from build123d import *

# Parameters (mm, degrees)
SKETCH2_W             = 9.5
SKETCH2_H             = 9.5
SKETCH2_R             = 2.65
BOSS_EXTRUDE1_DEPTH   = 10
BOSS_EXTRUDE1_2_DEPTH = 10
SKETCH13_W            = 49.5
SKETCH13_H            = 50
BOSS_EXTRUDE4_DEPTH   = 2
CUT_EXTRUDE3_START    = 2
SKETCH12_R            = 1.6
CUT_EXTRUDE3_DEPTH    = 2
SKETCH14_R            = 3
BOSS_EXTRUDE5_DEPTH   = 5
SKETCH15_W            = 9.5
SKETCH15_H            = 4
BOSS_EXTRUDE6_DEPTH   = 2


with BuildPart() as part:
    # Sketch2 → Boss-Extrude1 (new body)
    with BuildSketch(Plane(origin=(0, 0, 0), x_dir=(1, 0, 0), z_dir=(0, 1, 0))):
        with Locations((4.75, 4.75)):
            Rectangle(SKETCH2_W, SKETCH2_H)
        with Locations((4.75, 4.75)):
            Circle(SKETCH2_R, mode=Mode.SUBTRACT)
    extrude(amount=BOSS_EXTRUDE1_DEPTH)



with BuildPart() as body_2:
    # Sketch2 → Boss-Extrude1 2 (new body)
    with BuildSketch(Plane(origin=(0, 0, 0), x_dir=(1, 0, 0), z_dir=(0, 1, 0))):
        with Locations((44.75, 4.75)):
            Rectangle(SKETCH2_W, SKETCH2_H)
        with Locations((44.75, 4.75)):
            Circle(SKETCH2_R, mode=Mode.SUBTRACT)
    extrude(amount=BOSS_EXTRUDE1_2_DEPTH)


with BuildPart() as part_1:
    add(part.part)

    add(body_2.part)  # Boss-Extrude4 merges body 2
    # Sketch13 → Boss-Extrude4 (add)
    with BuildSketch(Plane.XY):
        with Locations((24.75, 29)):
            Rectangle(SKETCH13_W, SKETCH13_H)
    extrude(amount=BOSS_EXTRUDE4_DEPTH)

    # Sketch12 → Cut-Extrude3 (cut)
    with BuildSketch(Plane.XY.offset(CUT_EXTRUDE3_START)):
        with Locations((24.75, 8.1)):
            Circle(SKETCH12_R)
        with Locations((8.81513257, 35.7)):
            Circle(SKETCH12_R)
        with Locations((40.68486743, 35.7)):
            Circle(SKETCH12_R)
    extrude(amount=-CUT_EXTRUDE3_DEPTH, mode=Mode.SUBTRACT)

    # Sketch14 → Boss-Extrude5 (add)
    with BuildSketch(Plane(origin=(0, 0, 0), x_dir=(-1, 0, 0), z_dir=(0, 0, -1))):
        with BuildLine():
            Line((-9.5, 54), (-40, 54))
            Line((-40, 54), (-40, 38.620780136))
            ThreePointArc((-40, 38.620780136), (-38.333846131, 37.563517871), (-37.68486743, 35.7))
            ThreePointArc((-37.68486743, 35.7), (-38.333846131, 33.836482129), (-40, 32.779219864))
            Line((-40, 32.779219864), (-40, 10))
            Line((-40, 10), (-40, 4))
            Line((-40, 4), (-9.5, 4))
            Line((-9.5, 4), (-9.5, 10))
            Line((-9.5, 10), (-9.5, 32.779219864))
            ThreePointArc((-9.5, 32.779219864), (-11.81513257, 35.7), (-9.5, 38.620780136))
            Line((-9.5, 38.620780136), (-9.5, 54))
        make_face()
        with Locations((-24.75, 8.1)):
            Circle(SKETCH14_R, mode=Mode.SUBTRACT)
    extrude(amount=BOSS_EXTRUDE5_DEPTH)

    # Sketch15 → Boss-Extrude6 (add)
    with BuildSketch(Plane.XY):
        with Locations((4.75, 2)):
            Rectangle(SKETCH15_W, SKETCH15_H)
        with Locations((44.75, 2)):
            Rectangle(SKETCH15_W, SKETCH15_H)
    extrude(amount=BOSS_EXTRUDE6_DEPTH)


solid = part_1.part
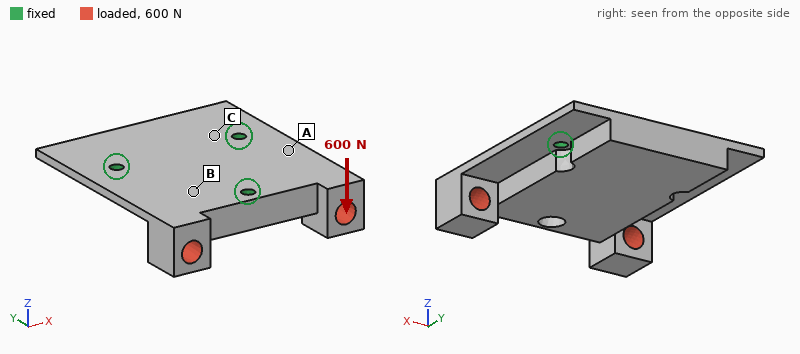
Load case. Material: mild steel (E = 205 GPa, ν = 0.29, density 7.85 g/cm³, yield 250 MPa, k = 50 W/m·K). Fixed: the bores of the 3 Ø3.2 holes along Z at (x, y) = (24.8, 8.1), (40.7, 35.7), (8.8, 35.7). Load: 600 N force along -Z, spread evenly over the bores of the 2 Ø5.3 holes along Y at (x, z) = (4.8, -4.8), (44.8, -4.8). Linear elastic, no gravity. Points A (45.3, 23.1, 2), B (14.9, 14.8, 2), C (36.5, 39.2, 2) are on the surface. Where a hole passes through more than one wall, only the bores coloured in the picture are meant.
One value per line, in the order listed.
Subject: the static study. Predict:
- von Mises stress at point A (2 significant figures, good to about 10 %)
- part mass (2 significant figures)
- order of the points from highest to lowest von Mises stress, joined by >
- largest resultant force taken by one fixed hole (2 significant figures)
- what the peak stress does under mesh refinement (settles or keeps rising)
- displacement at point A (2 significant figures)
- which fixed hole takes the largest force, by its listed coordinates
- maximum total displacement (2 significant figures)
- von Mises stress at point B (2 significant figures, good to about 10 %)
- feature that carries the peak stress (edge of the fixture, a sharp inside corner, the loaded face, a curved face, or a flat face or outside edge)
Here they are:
13 MPa
110 g
B > A > C
660 N
keeps rising
3.5 µm
(24.8, 8.1)
19 µm
25 MPa
edge of the fixture
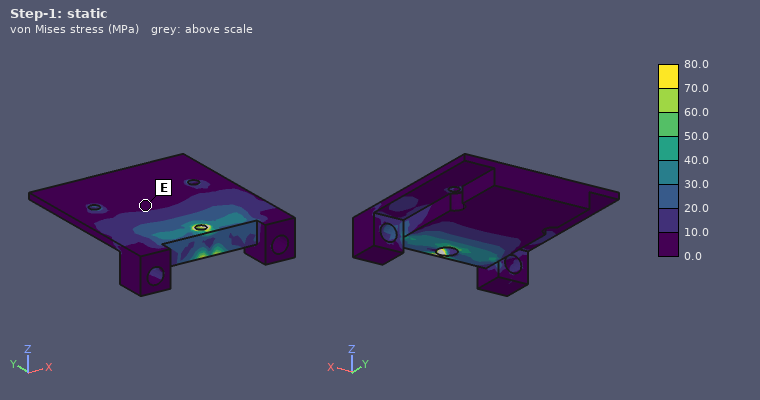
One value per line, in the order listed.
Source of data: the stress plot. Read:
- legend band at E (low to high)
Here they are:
0.0 to 10.0 MPa
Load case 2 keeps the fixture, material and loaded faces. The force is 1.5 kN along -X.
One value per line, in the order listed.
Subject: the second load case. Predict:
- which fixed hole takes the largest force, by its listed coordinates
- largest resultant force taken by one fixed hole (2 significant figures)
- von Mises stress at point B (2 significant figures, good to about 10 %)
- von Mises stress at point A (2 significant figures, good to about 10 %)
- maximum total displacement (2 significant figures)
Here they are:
(24.8, 8.1)
1.0 kN
19 MPa
21 MPa
23 µm
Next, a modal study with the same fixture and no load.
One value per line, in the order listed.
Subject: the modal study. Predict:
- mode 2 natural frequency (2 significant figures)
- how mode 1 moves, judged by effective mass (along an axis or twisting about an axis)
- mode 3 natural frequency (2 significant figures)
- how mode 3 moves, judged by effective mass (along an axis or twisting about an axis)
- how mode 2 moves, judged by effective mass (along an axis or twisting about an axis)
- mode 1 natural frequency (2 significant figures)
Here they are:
7500 Hz
twisting about Y
8900 Hz
along Z
twisting about X
6000 Hz
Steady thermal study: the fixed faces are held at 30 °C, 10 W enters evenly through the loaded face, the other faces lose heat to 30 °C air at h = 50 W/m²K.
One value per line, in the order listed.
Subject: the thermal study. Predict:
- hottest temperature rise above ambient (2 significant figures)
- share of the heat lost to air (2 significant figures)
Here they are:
27 K
29 %
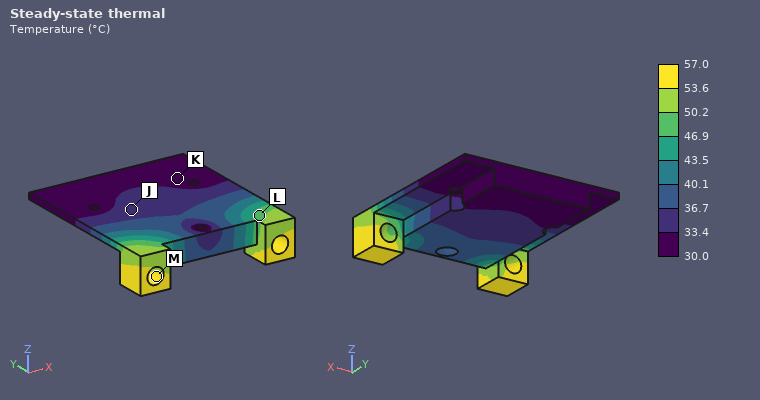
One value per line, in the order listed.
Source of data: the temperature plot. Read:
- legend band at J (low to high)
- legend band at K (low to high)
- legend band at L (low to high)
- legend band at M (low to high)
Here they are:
33.4 to 36.7 °C
30.0 to 33.4 °C
46.9 to 50.2 °C
53.6 to 57.0 °C
